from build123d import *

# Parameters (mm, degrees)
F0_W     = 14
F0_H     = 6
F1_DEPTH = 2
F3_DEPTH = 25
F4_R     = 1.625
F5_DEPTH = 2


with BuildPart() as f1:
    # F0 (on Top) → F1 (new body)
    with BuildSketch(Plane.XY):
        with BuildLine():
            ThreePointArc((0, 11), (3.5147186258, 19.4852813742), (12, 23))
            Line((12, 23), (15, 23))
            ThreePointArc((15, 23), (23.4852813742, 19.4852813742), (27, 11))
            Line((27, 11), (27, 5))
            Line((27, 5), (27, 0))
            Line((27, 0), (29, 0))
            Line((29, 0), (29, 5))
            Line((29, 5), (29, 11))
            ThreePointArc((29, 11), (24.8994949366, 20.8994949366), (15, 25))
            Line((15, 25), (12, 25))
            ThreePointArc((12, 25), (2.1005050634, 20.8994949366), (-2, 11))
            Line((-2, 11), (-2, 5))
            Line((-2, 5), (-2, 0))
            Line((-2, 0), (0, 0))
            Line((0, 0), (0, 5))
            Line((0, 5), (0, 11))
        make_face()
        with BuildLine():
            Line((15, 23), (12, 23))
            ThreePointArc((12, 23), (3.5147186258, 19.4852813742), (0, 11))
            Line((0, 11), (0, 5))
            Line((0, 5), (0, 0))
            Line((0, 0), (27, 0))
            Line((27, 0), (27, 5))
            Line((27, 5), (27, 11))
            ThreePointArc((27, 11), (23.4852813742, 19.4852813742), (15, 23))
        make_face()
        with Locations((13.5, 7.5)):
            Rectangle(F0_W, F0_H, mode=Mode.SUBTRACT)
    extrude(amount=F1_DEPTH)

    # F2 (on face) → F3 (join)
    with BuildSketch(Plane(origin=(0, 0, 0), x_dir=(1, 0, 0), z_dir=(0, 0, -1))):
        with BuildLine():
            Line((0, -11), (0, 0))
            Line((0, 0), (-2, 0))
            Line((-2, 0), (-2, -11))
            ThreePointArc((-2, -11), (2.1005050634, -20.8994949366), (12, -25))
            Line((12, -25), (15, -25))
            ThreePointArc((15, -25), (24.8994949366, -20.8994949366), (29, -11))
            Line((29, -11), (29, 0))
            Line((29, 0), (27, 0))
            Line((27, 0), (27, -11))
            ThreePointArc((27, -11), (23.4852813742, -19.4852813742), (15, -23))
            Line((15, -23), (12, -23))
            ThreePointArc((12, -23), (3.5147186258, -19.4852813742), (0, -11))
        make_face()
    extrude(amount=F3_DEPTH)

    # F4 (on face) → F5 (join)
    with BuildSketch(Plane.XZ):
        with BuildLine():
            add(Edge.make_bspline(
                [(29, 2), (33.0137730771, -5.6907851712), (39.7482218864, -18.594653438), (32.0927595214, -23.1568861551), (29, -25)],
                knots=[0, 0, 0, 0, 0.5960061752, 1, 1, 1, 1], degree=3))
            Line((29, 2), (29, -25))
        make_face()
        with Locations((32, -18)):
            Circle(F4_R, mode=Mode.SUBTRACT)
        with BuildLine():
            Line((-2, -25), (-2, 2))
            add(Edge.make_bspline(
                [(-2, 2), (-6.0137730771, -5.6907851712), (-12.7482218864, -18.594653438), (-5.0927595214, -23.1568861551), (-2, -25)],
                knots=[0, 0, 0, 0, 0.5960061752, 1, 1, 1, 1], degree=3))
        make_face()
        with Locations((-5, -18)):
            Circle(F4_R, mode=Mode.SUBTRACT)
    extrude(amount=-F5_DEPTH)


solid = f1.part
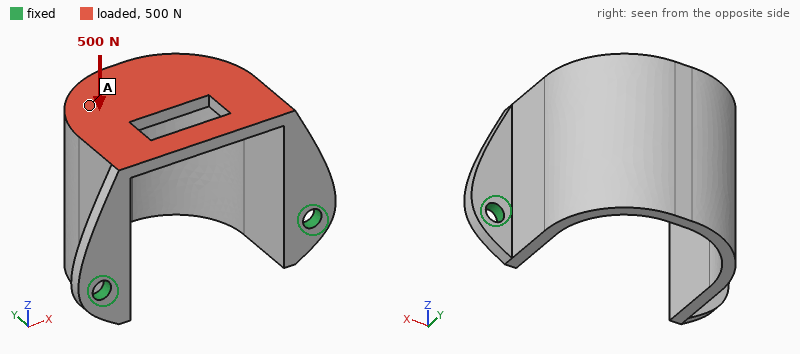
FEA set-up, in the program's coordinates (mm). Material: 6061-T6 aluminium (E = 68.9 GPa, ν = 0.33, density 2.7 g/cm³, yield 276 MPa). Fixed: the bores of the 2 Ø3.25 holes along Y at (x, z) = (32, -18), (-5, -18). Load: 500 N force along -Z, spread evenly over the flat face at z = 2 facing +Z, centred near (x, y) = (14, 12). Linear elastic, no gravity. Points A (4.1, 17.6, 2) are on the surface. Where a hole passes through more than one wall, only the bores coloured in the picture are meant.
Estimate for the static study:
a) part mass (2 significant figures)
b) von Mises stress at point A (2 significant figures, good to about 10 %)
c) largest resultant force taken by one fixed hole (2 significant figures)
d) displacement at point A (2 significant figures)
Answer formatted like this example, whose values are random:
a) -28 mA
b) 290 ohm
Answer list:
a) 13 g
b) 19 MPa
c) 260 N
d) 0.19 mm
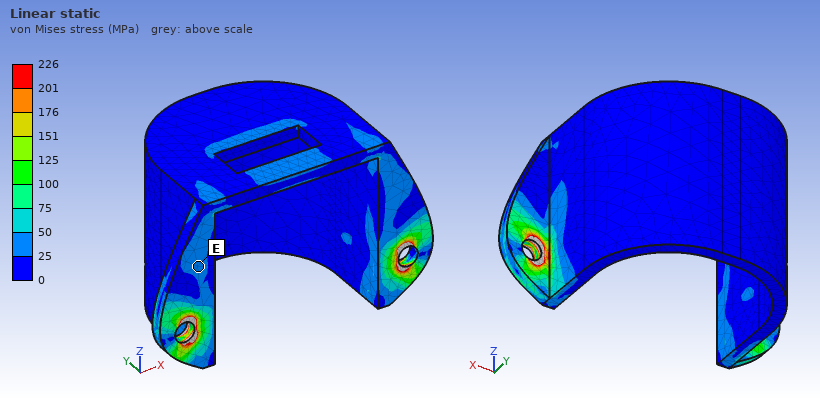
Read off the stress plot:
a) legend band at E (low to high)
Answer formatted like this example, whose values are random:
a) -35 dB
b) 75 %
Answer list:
a) 25 to 50 MPa
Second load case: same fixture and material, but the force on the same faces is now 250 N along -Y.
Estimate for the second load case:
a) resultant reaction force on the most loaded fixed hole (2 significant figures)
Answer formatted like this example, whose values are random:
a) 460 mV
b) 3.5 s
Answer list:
a) 130 N
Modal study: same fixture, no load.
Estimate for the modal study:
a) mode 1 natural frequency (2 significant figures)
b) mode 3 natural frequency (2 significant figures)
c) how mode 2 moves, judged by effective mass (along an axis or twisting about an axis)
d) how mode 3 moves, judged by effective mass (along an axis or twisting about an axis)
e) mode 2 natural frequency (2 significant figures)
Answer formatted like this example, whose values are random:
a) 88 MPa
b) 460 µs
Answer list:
a) 2000 Hz
b) 6600 Hz
c) along X
d) along X
e) 3500 Hz
